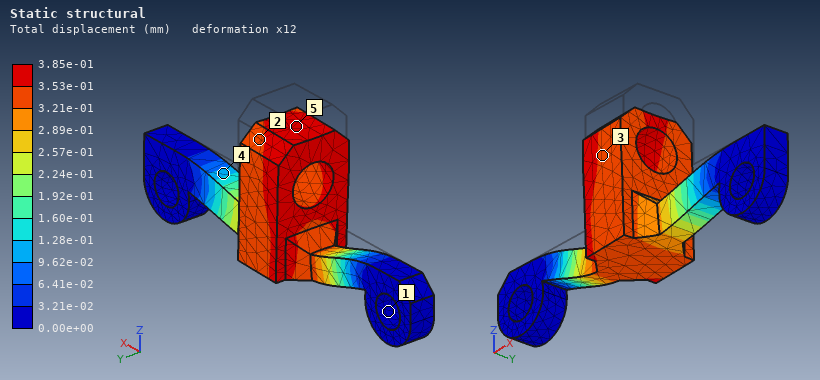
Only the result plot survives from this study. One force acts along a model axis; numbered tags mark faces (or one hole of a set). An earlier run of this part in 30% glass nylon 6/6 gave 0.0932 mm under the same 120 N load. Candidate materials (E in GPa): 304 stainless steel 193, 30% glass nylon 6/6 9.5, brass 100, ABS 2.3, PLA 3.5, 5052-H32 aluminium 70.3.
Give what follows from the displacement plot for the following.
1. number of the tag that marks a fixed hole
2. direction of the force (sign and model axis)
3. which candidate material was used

1
-Z
ABS
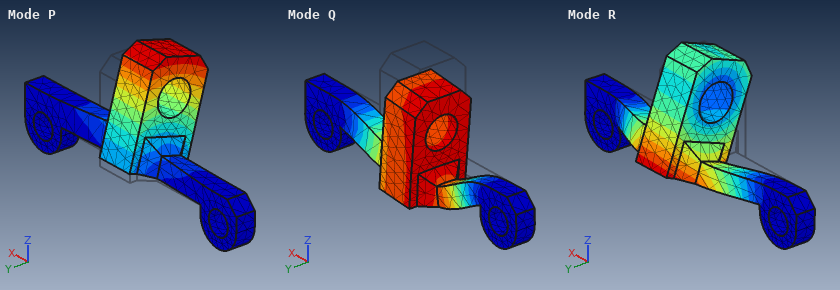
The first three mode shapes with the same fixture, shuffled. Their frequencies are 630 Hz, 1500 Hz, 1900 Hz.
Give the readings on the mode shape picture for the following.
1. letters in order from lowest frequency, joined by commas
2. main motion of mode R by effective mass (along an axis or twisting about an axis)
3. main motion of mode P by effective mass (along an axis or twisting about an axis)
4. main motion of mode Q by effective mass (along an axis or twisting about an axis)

P, Q, R
along Y
along Y
along Z
